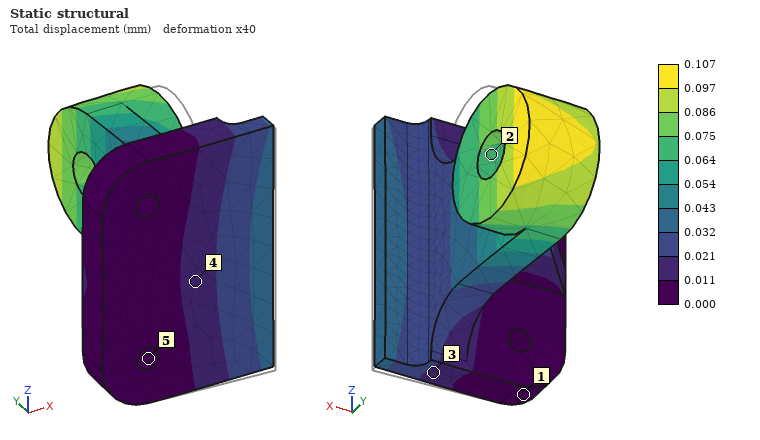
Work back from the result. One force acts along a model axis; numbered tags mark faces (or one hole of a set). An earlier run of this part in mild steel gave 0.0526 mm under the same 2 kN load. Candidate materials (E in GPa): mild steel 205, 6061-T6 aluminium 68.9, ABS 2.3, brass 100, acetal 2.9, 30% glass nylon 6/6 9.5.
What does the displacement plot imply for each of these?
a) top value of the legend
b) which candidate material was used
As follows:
0.107 mm
brass
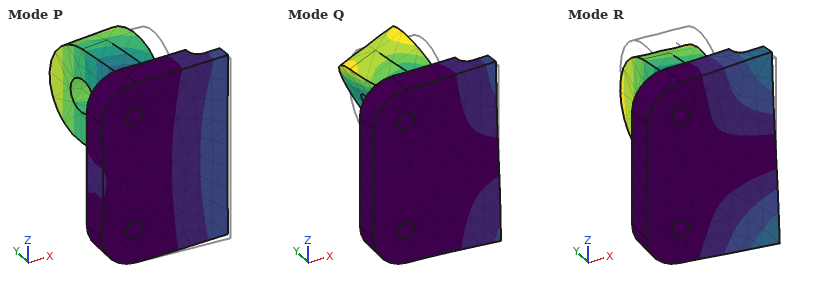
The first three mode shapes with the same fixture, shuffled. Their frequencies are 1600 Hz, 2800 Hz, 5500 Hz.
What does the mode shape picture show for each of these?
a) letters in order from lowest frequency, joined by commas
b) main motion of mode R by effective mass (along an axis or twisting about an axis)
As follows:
P, R, Q
along Z
